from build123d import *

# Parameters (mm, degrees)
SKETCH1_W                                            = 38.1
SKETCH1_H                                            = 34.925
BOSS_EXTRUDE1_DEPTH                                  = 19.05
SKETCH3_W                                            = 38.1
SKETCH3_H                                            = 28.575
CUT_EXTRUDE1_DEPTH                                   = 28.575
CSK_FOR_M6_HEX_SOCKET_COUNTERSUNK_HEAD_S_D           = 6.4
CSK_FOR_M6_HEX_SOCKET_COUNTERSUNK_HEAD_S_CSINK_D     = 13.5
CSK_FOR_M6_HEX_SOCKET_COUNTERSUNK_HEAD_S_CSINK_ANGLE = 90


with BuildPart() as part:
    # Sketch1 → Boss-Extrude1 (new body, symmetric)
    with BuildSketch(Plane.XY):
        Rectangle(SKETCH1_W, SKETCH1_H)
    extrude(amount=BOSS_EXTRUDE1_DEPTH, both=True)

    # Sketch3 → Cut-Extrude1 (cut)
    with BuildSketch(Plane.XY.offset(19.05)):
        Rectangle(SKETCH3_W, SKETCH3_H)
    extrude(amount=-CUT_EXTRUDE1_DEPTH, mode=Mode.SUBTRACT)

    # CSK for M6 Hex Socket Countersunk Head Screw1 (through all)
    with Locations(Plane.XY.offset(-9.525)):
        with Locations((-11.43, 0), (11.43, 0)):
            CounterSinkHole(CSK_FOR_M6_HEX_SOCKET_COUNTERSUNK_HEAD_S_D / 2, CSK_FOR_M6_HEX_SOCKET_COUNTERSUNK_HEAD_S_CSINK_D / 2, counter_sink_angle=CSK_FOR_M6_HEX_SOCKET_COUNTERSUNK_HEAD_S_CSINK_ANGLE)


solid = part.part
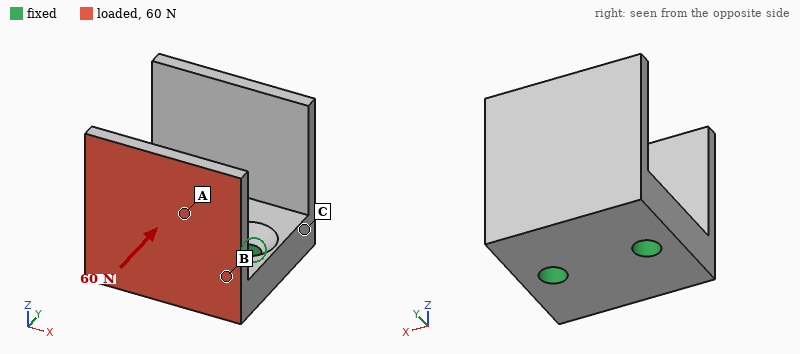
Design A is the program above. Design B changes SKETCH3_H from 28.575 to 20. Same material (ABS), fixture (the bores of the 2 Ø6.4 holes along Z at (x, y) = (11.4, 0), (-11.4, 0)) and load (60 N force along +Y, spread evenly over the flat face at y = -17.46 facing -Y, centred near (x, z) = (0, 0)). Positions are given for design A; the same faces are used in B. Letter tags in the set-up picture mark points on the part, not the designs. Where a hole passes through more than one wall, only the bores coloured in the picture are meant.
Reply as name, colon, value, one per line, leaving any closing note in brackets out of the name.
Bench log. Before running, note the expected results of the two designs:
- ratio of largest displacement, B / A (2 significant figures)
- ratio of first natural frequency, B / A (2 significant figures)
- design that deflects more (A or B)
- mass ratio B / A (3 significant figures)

ratio of largest displacement, B / A: 0.20
ratio of first natural frequency, B / A: 1.3
design that deflects more: A
mass ratio B / A: 1.50
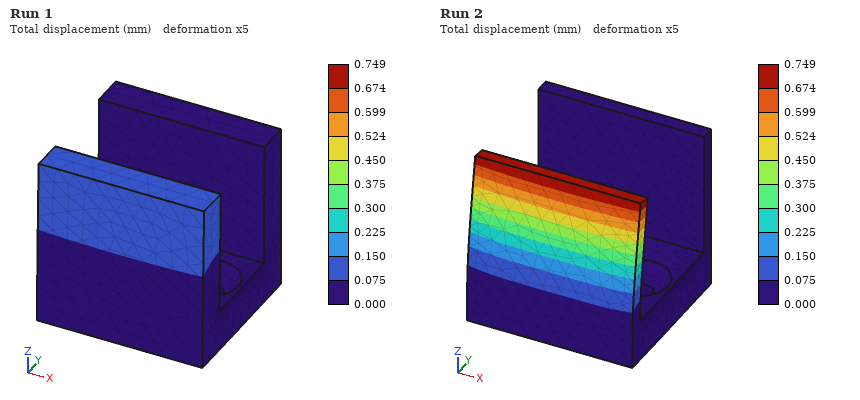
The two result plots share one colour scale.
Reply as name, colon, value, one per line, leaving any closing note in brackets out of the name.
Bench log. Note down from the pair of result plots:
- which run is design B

which run is design B: Run 1
